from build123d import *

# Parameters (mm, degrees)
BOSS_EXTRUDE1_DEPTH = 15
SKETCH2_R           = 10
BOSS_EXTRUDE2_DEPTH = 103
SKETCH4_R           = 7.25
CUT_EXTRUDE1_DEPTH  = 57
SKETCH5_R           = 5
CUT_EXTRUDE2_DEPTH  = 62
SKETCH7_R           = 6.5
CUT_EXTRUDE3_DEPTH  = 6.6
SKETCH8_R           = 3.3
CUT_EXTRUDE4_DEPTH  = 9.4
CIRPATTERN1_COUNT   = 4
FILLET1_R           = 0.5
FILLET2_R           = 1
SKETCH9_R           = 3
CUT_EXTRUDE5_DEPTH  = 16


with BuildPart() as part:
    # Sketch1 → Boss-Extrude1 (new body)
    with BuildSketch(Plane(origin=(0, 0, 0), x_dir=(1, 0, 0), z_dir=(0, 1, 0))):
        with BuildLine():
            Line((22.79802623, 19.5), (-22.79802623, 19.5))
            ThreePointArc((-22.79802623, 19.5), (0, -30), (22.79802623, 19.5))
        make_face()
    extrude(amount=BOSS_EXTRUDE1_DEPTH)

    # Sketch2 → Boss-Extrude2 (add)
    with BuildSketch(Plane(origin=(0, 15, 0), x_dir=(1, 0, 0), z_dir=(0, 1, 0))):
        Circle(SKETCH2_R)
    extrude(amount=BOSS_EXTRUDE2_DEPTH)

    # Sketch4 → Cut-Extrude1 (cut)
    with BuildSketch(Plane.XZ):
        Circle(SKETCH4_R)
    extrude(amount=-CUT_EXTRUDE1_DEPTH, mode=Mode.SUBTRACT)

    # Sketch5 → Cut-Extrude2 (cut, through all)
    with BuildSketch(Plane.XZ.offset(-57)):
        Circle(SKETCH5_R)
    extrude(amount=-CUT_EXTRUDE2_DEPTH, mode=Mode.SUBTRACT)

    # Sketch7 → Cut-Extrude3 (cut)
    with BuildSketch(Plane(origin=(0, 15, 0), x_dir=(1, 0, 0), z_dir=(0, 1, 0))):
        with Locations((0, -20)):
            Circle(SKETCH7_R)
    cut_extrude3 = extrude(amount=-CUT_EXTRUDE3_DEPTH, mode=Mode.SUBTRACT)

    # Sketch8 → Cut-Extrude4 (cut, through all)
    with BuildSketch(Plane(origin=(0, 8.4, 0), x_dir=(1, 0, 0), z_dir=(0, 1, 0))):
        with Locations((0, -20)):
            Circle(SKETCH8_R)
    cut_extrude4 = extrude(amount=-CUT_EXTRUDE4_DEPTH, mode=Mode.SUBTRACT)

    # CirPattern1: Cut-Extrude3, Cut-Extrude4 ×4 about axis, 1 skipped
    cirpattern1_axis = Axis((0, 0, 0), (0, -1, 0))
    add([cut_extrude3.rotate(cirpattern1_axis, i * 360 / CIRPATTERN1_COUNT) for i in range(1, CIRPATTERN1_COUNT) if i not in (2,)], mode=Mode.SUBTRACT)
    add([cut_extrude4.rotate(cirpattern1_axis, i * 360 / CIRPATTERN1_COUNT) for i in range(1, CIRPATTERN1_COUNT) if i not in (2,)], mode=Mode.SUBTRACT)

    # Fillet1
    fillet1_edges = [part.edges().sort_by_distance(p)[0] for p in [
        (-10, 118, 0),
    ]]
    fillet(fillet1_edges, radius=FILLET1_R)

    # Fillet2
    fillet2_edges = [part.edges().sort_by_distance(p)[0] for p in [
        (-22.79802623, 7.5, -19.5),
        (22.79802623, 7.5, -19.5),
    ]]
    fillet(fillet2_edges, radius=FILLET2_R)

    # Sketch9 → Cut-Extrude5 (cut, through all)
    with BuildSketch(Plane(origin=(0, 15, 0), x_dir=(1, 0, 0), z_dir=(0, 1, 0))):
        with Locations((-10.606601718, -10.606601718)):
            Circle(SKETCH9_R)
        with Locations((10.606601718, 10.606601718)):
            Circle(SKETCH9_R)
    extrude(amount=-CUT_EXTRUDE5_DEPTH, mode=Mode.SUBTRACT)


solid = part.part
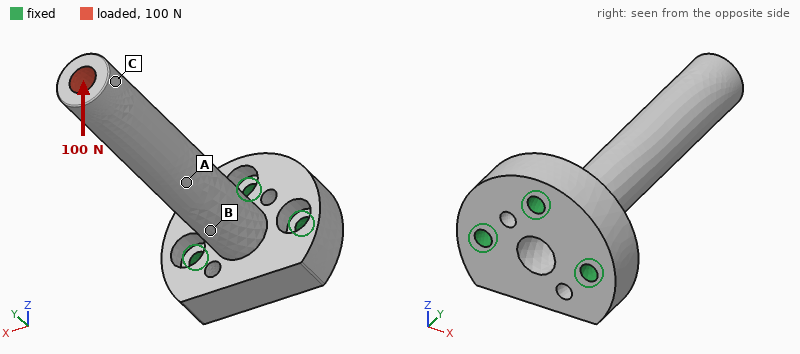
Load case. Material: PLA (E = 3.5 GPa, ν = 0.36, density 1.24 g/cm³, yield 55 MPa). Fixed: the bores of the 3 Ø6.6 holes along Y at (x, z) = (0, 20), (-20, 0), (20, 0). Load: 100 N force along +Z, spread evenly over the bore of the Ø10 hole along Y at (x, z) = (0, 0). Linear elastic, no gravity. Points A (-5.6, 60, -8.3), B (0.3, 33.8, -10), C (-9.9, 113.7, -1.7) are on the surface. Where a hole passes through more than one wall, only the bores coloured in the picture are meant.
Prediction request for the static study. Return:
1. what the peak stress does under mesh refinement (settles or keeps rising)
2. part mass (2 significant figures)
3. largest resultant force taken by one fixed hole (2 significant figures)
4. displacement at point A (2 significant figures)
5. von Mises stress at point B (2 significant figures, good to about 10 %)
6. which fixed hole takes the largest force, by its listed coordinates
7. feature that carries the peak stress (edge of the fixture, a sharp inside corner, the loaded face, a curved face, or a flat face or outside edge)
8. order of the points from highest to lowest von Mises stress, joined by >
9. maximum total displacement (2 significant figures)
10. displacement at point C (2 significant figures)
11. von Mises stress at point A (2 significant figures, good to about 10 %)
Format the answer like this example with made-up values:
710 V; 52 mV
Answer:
keeps rising; 64 g; 300 N; 0.50 mm; 9.7 MPa; (0, 20); a sharp inside corner; B > A > C; 1.4 mm; 1.4 mm; 3.5 MPa
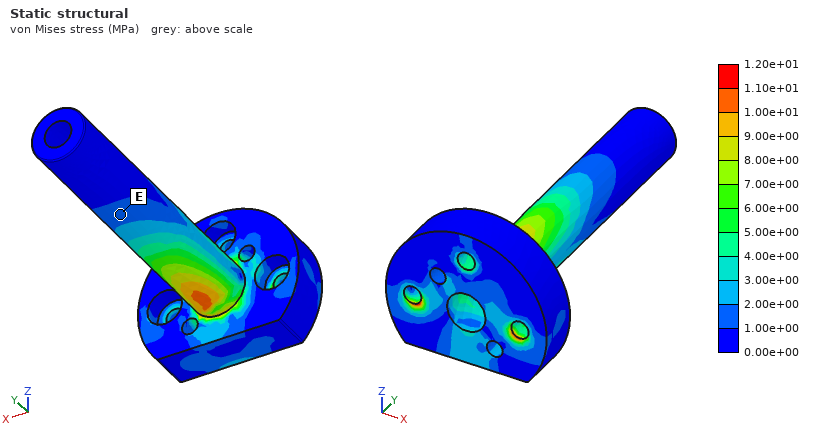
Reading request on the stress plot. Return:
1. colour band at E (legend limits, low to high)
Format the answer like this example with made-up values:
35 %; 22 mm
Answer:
1.00e+00 to 2.00e+00 MPa
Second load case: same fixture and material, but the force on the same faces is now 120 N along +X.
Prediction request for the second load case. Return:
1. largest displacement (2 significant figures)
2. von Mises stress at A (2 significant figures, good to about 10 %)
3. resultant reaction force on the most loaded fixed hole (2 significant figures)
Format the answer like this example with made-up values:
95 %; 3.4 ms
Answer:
1.6 mm; 3.1 MPa; 290 N
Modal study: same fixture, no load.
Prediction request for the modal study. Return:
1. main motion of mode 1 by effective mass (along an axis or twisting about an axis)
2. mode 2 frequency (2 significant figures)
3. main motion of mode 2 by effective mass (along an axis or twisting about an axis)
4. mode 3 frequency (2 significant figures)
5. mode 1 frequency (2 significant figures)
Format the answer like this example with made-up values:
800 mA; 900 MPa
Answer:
along Z; 390 Hz; along X; 2200 Hz; 370 Hz
